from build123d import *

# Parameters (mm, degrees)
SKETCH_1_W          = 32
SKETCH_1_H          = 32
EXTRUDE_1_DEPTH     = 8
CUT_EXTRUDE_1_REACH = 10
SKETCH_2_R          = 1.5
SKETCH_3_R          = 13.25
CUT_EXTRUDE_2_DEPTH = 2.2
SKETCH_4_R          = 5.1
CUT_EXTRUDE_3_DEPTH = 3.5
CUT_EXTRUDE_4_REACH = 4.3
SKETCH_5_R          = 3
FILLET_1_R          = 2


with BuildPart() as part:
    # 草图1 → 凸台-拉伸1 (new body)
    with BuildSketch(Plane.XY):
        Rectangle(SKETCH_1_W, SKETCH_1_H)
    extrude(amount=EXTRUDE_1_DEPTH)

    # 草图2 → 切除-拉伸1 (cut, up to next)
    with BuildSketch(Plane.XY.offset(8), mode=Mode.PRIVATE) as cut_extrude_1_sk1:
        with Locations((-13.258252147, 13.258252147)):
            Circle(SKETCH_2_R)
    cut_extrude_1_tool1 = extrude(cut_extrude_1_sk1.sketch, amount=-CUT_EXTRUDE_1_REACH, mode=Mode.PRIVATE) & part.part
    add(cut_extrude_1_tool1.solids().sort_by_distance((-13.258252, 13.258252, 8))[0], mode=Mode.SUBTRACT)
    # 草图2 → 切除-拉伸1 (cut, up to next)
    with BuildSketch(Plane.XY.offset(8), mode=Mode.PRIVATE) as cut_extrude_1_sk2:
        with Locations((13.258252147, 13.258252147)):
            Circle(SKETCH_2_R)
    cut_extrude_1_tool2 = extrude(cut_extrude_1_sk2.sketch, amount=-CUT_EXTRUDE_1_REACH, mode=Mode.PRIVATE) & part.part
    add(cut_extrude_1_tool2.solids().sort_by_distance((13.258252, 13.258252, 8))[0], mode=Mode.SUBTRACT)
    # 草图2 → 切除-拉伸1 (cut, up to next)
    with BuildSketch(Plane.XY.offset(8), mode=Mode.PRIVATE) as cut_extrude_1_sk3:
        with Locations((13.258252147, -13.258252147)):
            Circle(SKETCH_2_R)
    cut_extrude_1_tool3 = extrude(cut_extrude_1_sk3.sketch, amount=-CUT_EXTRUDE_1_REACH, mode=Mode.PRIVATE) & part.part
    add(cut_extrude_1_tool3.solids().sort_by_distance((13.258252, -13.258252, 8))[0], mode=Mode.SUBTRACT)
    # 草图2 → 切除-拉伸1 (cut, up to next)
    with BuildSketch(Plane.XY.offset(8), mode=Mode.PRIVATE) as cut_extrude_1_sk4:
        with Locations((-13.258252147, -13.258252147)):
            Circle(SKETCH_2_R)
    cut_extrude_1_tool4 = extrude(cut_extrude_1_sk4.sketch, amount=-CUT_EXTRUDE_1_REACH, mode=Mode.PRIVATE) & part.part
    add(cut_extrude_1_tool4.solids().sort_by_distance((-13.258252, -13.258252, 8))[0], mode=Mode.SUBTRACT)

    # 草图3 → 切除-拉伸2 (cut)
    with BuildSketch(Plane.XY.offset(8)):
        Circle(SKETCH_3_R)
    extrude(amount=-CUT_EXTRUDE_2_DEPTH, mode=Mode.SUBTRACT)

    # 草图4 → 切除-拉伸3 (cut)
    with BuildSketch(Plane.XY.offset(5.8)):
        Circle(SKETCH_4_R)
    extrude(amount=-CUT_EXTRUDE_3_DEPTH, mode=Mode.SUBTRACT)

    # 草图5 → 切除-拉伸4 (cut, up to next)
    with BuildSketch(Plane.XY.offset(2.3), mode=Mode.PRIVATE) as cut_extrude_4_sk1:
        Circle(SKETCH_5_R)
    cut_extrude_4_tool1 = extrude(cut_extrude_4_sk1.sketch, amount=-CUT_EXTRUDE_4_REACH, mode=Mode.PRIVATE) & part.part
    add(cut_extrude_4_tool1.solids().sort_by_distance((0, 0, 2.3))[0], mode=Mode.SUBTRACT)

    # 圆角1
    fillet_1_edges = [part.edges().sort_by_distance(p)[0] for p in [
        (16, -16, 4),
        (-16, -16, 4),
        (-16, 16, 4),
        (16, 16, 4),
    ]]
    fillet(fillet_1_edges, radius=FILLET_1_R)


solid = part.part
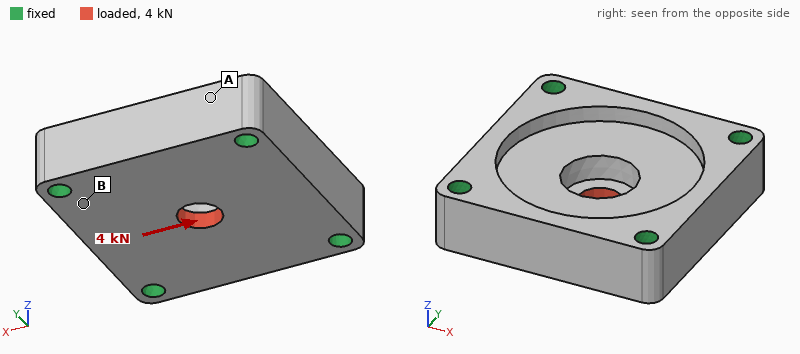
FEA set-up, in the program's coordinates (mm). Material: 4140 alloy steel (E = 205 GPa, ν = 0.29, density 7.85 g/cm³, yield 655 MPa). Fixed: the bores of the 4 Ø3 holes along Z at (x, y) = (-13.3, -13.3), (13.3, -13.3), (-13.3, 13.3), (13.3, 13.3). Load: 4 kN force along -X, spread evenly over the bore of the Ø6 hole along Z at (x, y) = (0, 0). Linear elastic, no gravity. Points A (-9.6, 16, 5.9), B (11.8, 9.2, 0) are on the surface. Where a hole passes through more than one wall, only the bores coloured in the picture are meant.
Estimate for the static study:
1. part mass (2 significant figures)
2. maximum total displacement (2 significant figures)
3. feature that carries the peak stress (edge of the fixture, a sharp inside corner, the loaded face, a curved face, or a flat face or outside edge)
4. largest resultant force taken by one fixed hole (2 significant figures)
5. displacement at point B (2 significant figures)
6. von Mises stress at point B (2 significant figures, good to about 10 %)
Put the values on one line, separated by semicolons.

50 g; 4.1 µm; a sharp inside corner; 1.1 kN; 0.69 µm; 26 MPa
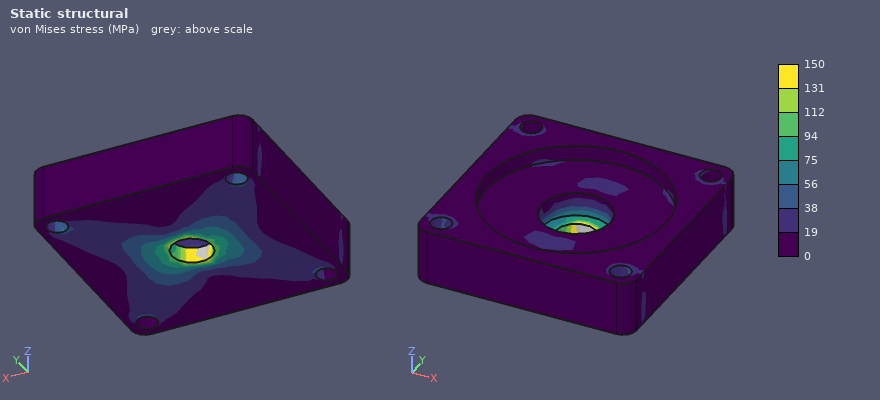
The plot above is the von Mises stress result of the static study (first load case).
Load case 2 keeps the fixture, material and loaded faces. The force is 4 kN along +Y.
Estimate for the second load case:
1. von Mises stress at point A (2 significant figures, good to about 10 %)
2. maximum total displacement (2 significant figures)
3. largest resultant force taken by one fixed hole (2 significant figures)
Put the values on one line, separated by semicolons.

11 MPa; 4.1 µm; 1.1 kN
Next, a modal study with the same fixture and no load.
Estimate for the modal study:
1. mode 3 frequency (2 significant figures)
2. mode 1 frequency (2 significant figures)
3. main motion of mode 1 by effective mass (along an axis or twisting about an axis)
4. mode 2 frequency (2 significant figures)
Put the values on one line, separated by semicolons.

43 kHz; 31 kHz; along Z; 43 kHz
